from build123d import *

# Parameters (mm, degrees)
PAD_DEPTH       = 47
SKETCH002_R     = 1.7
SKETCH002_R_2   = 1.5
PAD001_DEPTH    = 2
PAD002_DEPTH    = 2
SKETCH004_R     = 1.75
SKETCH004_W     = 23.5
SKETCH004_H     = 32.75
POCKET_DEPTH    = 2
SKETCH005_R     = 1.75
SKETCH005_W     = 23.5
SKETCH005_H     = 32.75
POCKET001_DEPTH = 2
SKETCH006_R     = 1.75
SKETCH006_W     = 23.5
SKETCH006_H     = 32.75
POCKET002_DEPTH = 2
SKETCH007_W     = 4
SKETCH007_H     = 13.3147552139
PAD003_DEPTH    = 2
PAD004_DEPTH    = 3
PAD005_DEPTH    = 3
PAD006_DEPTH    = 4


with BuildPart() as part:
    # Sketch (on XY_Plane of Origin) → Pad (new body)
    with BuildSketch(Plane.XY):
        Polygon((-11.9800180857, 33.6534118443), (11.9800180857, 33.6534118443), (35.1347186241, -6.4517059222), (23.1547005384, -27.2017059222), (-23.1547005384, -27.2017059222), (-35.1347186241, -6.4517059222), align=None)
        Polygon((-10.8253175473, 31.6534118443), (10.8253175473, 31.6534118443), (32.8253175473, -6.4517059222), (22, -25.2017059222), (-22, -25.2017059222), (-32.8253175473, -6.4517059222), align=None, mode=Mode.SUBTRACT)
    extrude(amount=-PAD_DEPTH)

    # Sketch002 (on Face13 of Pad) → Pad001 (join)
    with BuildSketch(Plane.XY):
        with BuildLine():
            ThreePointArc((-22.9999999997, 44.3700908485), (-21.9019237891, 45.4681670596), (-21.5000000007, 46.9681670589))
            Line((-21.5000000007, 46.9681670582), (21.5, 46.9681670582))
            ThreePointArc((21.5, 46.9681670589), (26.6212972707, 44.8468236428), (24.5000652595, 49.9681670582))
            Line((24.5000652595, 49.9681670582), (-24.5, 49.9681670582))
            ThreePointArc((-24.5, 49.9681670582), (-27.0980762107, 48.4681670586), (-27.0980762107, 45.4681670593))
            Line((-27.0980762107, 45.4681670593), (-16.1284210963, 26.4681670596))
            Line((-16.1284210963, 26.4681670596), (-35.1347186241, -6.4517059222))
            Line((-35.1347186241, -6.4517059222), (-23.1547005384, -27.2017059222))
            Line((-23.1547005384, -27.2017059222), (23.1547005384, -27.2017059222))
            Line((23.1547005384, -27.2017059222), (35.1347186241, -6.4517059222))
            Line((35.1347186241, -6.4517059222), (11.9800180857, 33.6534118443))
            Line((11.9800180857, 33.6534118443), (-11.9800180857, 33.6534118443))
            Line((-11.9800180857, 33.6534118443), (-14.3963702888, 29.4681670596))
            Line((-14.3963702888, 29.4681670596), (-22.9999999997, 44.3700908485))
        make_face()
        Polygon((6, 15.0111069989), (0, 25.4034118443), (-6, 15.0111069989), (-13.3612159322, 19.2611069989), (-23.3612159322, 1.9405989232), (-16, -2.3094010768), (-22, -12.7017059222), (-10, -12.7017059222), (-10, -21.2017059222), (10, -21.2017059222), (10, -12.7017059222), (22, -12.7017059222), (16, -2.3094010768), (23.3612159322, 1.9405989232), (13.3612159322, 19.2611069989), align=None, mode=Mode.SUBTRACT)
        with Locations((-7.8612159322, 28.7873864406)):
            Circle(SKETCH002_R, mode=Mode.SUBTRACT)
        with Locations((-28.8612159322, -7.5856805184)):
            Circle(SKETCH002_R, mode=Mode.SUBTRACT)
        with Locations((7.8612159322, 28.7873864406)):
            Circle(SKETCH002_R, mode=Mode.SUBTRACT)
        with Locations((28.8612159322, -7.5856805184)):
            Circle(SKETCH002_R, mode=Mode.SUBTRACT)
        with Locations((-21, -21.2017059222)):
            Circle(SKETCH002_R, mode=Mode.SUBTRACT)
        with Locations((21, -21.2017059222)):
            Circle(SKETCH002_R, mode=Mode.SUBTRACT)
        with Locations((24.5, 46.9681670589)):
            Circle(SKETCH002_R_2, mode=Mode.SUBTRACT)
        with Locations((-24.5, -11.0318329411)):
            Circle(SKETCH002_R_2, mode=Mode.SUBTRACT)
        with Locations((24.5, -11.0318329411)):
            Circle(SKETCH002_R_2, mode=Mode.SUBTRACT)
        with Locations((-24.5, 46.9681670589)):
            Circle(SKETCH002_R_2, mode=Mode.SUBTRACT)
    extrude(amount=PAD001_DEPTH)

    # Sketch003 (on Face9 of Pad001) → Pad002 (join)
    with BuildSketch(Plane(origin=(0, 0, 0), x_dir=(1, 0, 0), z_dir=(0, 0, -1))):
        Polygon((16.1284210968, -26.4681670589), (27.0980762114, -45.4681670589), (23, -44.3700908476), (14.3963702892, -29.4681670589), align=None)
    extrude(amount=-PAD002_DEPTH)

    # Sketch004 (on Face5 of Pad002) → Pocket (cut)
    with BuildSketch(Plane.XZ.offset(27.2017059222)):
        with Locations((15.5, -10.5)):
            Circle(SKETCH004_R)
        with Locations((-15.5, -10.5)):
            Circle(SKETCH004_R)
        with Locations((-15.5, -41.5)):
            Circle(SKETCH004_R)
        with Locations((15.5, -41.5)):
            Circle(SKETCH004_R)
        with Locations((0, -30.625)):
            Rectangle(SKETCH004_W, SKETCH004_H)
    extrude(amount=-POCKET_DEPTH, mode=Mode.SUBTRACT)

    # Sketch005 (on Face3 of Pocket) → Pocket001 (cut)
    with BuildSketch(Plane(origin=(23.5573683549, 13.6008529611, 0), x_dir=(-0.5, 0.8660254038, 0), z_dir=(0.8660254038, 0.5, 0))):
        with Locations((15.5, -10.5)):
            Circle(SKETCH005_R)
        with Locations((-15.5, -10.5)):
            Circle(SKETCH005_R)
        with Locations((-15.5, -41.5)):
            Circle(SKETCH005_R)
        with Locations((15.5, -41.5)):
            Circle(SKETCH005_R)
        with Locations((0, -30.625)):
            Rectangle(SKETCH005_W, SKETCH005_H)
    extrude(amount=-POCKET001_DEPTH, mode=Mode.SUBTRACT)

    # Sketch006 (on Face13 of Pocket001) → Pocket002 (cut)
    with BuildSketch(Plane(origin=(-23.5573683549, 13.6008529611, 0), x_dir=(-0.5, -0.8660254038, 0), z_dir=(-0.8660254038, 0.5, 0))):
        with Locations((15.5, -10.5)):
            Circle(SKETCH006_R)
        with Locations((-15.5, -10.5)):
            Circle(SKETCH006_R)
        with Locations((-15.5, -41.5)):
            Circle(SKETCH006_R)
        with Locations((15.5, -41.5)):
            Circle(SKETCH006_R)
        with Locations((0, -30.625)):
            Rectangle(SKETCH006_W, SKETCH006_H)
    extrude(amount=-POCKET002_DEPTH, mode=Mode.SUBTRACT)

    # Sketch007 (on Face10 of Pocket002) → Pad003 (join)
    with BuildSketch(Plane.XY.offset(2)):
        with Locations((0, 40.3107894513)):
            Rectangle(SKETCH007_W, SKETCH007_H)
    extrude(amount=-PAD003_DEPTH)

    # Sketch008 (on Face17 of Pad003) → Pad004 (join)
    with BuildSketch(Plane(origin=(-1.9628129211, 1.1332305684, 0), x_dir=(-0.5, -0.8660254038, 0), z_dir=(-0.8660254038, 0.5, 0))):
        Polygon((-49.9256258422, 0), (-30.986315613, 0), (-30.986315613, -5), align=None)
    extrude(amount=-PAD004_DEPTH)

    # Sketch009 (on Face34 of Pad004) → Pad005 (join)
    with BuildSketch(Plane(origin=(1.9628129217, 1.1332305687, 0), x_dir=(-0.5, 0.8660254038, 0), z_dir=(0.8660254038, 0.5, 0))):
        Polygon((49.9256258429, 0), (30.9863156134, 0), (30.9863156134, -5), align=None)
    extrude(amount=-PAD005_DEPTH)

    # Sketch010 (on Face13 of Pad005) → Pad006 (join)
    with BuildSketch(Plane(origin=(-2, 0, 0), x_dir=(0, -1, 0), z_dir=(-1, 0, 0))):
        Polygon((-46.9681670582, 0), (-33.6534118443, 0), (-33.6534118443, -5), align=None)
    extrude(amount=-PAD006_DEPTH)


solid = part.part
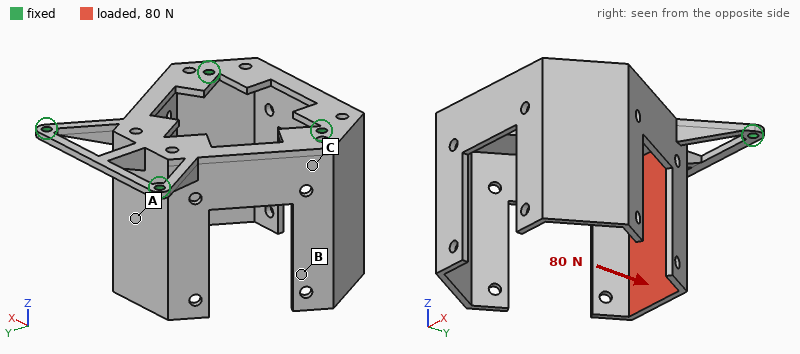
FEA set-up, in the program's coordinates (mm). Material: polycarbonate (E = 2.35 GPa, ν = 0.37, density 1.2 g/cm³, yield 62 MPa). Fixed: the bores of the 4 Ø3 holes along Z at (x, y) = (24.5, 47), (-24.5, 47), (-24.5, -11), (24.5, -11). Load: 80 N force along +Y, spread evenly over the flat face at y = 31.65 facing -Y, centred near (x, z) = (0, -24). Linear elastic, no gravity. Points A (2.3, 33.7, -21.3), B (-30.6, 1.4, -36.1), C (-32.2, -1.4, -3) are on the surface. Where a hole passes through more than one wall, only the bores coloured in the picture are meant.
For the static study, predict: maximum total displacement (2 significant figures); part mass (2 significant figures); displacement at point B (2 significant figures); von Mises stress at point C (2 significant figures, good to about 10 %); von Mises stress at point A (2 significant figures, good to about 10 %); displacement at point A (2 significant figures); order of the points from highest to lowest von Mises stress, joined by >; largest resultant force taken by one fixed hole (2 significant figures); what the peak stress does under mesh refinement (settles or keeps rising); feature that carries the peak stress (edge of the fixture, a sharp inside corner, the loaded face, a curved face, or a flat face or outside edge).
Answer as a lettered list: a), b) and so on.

a) 1.3 mm
b) 23 g
c) 0.53 mm
d) 2.3 MPa
e) 5.7 MPa
f) 0.68 mm
g) A > C > B
h) 33 N
i) keeps rising
j) edge of the fixture
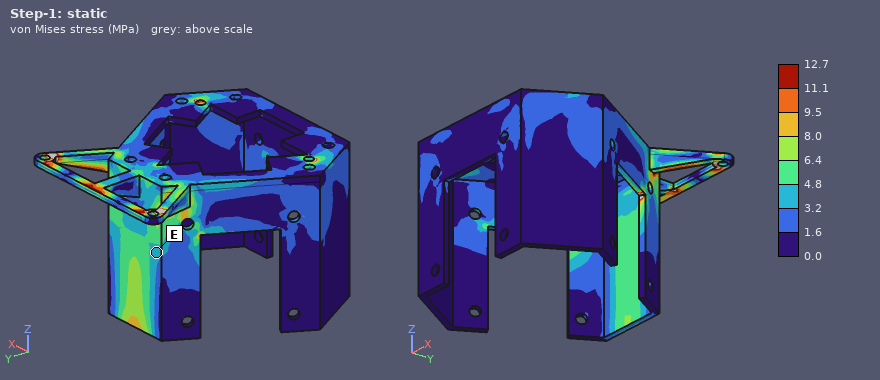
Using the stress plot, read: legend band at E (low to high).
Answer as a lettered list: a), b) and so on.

a) 3.2 to 4.8 MPa
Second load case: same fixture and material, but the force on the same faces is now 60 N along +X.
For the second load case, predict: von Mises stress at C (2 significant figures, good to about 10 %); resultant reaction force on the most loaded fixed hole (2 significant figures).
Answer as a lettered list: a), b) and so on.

a) 1.5 MPa
b) 40 N
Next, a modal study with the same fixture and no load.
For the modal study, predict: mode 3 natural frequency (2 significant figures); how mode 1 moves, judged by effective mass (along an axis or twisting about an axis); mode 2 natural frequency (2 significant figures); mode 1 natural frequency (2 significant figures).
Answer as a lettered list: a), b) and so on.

a) 530 Hz
b) along Y
c) 420 Hz
d) 320 Hz
